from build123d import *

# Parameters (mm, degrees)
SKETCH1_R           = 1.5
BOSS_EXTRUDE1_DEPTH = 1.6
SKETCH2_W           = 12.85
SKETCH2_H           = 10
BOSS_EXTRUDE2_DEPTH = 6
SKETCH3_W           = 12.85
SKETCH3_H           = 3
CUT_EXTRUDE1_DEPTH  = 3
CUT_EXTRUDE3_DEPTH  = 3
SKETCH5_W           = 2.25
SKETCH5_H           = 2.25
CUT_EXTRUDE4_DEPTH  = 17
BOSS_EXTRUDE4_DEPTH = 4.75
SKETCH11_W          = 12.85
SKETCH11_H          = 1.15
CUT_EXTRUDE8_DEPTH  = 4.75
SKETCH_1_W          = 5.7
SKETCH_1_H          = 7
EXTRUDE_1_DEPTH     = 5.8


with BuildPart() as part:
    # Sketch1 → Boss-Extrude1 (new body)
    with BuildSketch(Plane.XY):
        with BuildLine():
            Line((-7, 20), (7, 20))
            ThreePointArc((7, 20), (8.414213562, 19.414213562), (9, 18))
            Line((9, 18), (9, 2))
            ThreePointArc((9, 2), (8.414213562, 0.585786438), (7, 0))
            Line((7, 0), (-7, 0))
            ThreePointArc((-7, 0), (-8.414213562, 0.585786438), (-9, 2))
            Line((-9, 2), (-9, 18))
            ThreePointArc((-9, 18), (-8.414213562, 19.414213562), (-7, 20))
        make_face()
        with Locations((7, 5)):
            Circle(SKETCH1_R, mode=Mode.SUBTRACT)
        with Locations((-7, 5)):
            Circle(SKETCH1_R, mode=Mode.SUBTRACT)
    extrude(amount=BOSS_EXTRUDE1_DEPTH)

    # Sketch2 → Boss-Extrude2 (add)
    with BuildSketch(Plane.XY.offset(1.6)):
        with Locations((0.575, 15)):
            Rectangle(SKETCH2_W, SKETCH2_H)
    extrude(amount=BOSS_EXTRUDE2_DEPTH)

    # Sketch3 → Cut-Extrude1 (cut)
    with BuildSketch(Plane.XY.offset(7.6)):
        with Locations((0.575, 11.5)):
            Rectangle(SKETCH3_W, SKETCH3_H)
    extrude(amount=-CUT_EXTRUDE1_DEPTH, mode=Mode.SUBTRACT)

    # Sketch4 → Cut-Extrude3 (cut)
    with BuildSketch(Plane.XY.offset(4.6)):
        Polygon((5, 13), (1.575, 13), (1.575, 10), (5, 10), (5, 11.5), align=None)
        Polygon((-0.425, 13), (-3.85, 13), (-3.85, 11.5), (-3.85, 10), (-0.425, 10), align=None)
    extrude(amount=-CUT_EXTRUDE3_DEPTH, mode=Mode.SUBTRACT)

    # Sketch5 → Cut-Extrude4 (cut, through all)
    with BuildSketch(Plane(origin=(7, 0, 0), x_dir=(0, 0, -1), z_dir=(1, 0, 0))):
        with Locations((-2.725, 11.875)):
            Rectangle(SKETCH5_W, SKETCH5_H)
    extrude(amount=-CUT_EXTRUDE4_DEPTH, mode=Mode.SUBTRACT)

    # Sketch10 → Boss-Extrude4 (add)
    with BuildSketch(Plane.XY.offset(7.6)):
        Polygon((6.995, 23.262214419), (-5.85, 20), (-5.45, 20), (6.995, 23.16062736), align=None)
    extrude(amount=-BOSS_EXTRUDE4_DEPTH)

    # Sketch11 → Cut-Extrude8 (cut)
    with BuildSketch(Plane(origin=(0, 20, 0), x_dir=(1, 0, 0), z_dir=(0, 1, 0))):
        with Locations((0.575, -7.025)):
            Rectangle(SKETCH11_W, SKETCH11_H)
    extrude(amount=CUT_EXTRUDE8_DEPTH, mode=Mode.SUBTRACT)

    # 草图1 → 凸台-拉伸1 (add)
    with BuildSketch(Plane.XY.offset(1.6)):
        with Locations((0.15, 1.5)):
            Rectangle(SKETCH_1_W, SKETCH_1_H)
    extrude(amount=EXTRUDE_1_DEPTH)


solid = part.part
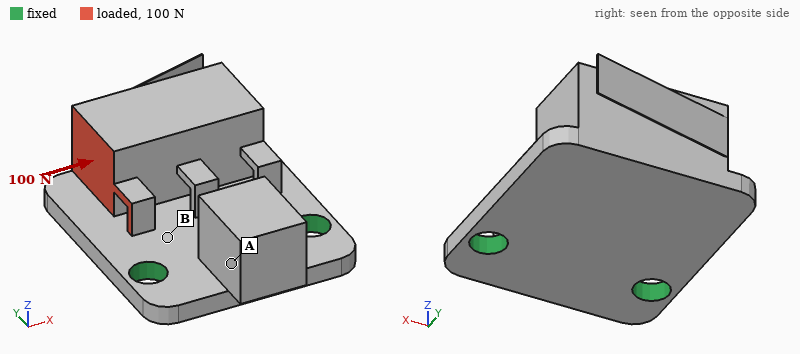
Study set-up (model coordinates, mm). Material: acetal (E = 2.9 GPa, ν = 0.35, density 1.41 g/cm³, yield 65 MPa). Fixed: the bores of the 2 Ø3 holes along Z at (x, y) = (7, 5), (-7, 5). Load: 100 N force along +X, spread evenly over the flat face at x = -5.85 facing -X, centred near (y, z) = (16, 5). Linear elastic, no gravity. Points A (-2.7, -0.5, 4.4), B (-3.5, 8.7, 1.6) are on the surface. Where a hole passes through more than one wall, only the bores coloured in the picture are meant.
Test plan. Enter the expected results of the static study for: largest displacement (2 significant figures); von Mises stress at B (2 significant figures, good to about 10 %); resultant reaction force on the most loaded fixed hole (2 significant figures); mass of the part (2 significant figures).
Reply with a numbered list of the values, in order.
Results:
1. 0.27 mm
2. 18 MPa
3. 92 N
4. 1.9 g
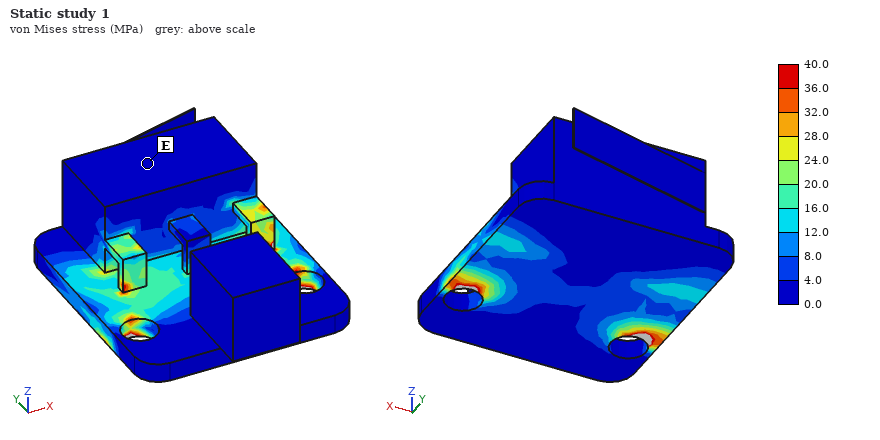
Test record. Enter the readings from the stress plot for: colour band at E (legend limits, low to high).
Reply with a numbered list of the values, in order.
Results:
1. 0.0 to 4.0 MPa
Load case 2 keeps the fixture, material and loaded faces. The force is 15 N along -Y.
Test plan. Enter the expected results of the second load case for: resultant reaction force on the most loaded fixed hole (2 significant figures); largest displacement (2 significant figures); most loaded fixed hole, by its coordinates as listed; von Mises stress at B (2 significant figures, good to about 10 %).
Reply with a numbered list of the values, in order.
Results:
1. 14 N
2. 0.31 mm
3. (-7, 5)
4. 6.9 MPa
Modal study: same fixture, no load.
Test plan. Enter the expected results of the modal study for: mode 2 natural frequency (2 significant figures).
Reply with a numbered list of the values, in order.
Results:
1. 920 Hz
